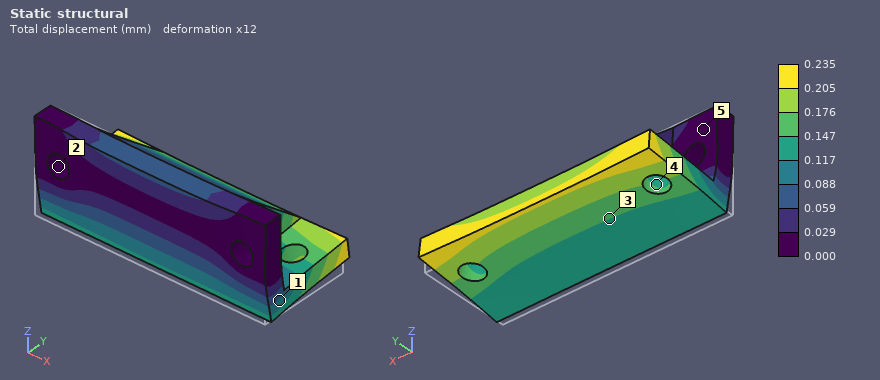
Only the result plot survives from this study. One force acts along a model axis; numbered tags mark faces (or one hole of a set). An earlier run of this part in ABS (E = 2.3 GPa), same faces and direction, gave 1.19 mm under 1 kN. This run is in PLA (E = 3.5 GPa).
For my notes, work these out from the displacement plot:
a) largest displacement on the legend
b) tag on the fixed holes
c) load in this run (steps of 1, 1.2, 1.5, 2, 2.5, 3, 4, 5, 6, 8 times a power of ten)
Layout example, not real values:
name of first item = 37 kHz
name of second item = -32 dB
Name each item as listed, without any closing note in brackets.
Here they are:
largest displacement on the legend = 0.235 mm
tag on the fixed holes = 2
load in this run = 300 N
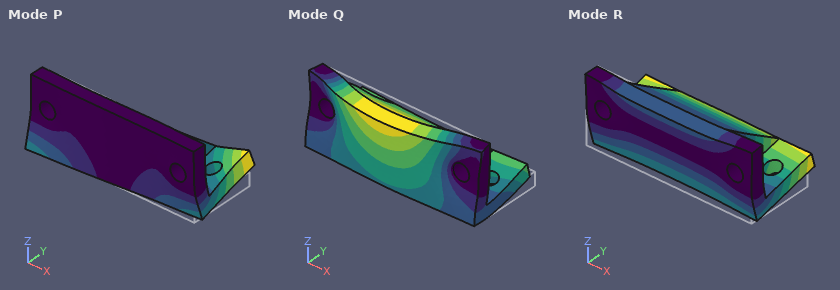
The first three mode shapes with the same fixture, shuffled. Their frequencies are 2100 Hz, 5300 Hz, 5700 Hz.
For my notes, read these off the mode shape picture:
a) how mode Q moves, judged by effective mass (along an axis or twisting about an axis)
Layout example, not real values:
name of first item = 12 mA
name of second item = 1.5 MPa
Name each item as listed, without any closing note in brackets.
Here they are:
how mode Q moves, judged by effective mass = along Y
